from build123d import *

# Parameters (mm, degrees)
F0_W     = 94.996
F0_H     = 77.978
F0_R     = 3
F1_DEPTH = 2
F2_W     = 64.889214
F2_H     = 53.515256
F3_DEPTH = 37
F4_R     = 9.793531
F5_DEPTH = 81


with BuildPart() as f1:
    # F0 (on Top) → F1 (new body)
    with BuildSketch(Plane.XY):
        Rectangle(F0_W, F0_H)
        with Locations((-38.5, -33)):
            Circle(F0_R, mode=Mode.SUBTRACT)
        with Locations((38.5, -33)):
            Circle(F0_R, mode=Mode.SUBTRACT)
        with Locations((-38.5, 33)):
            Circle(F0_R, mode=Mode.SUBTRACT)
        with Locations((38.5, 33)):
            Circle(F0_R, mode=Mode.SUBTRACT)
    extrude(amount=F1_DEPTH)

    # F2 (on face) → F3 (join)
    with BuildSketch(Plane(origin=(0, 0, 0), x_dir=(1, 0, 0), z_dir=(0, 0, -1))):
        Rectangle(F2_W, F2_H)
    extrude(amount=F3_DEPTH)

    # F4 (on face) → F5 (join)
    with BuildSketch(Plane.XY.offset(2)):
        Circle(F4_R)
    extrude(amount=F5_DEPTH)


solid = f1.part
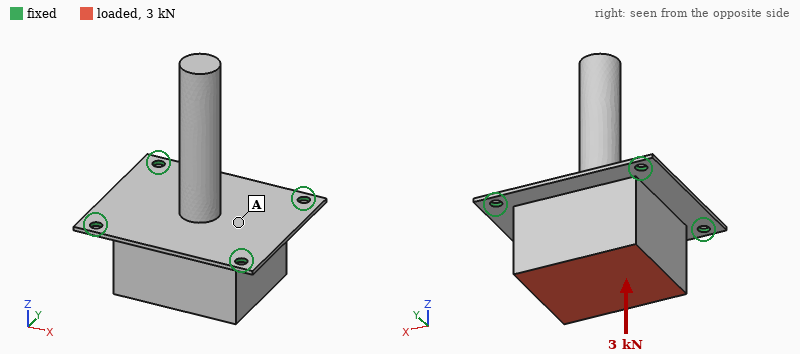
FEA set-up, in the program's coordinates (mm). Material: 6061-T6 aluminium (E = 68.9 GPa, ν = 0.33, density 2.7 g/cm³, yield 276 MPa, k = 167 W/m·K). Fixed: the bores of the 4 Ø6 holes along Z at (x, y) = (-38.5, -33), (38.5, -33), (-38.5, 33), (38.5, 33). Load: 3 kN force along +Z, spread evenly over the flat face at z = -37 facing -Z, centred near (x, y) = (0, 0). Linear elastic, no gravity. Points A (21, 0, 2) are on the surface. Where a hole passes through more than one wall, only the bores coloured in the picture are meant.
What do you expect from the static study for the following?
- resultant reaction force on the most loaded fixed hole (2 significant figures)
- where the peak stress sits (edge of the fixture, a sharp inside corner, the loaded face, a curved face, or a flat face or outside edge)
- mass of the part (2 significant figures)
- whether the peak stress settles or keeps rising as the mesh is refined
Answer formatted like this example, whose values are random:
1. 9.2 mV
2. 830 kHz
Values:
1. 860 N
2. edge of the fixture
3. 450 g
4. keeps rising
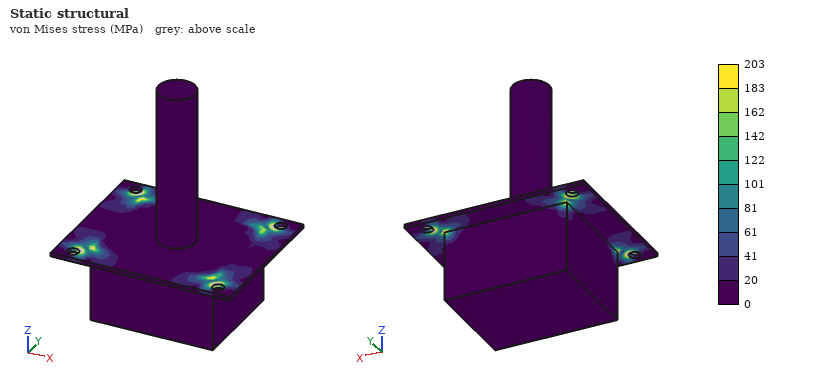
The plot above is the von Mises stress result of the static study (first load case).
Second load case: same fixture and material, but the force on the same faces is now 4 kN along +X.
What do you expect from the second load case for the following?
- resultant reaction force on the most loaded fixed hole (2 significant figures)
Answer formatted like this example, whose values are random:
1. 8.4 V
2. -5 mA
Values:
1. 1.6 kN
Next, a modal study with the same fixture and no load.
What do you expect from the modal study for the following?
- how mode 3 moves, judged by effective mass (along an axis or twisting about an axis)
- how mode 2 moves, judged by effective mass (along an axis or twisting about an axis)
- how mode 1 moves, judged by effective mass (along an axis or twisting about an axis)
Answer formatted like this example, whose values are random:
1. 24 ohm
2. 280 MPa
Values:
1. along Z
2. twisting about Y
3. twisting about X
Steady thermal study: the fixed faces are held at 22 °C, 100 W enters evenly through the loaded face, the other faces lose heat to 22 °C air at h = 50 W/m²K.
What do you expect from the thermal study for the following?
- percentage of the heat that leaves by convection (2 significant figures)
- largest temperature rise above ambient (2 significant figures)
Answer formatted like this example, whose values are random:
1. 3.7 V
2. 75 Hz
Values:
1. 34 %
2. 37 K
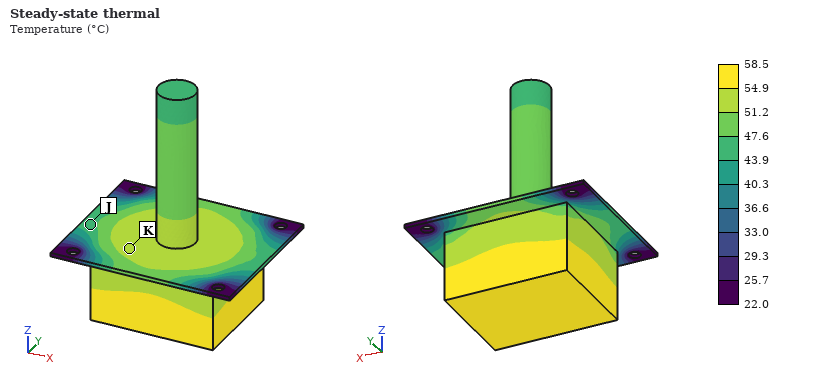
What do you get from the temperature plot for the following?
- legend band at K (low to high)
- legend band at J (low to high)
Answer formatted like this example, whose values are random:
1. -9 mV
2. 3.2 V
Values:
1. 51.2 to 54.9 °C
2. 43.9 to 47.6 °C
